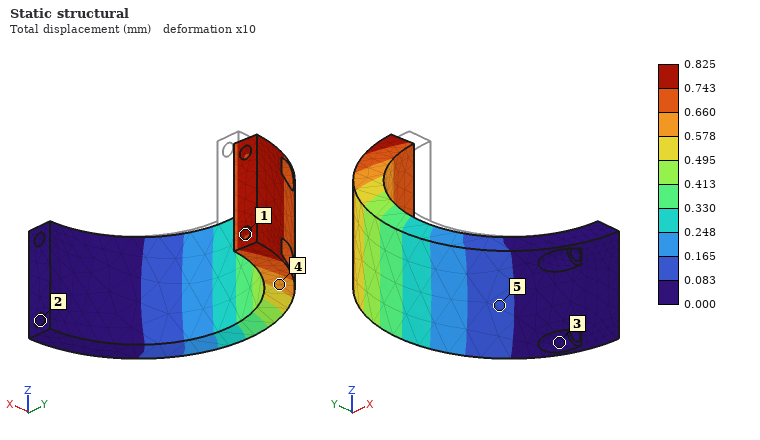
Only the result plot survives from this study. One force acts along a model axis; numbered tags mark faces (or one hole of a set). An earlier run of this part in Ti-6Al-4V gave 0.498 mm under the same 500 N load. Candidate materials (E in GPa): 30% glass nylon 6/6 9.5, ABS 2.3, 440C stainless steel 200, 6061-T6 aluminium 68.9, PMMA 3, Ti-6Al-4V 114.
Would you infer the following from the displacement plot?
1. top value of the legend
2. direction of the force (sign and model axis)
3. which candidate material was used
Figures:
0.825 mm
-X
6061-T6 aluminium
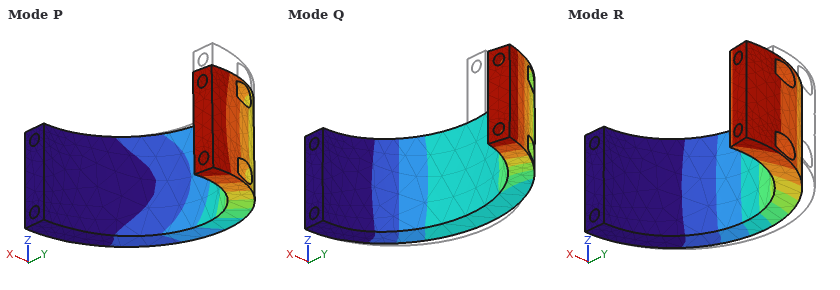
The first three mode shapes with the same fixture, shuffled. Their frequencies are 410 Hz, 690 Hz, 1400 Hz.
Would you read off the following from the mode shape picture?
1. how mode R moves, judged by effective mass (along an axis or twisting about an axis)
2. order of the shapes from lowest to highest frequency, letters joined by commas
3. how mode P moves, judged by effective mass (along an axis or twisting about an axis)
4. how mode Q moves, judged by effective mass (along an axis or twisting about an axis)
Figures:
along X
R, P, Q
along Z
along Y
